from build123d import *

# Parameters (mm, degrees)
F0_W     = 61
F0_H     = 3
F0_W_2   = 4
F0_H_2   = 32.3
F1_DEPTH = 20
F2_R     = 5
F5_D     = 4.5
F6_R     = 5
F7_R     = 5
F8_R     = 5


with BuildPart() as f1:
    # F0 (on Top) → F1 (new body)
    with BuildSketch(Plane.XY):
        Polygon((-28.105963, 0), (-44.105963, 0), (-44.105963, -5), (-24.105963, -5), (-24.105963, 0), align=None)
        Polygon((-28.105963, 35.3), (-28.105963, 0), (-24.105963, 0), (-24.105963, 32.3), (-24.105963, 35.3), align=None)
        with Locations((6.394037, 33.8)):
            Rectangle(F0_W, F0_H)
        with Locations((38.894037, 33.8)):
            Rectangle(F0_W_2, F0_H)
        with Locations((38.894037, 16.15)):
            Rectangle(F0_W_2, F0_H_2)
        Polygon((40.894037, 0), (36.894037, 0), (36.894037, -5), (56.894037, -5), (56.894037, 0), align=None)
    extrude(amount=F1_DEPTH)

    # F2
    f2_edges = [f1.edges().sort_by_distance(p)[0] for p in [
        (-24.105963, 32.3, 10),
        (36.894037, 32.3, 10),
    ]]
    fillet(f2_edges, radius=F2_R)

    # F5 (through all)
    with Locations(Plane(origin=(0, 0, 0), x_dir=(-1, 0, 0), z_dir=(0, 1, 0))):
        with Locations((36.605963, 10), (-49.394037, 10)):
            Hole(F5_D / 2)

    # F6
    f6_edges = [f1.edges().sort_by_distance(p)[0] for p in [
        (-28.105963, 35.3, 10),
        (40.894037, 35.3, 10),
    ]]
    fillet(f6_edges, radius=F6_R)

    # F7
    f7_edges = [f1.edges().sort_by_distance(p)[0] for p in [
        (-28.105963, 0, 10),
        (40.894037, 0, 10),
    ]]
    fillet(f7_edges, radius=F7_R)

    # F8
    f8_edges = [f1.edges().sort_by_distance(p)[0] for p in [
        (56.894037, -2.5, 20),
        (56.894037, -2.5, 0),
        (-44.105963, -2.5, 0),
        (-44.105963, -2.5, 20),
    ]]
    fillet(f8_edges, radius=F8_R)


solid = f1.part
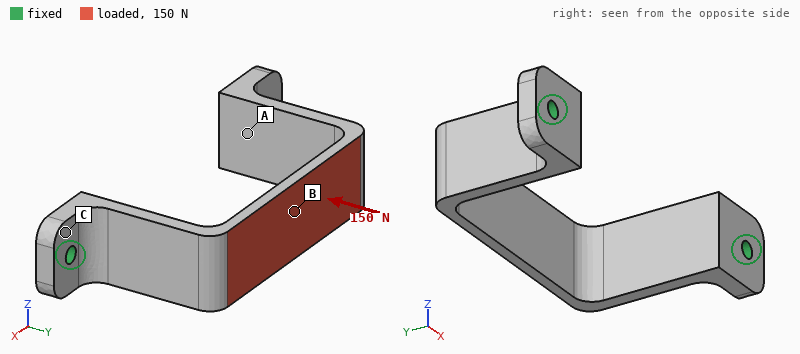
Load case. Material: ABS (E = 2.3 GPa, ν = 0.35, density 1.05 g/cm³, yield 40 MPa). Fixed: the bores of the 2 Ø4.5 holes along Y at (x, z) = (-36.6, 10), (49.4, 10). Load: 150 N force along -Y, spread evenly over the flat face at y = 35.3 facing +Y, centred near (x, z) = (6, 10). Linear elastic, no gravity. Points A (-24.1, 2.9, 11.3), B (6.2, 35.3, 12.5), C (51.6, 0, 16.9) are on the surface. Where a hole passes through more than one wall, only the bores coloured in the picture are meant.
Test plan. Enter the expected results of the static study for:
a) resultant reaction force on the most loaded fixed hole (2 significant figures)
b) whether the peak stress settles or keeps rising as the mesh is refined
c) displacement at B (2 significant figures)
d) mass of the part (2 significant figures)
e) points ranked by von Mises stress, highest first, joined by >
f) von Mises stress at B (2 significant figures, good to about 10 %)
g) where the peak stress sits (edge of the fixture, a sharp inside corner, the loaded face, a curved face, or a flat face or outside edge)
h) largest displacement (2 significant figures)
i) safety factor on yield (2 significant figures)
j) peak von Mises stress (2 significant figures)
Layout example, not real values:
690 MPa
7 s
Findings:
85 N
settles
1.1 mm
14 g
B > A > C
14 MPa
a curved face
1.1 mm
2.6
15 MPa
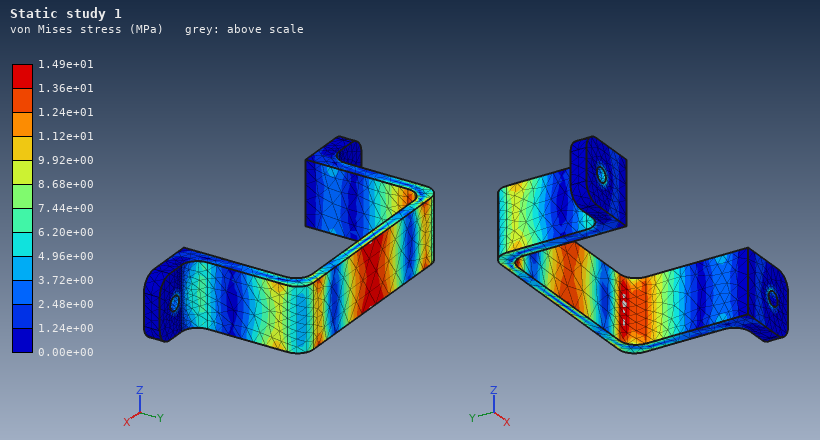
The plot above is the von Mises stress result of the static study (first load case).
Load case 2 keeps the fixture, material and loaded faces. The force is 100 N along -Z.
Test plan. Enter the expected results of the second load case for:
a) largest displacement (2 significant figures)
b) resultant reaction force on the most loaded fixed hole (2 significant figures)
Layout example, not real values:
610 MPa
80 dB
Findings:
1.1 mm
50 N
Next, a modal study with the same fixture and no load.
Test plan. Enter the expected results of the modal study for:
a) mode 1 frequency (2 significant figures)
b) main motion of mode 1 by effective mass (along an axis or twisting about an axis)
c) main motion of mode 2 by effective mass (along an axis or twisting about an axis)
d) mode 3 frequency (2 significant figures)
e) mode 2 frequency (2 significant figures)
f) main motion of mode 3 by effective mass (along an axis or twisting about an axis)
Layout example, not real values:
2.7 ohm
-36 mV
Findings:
530 Hz
along X
along Z
980 Hz
680 Hz
twisting about Y
